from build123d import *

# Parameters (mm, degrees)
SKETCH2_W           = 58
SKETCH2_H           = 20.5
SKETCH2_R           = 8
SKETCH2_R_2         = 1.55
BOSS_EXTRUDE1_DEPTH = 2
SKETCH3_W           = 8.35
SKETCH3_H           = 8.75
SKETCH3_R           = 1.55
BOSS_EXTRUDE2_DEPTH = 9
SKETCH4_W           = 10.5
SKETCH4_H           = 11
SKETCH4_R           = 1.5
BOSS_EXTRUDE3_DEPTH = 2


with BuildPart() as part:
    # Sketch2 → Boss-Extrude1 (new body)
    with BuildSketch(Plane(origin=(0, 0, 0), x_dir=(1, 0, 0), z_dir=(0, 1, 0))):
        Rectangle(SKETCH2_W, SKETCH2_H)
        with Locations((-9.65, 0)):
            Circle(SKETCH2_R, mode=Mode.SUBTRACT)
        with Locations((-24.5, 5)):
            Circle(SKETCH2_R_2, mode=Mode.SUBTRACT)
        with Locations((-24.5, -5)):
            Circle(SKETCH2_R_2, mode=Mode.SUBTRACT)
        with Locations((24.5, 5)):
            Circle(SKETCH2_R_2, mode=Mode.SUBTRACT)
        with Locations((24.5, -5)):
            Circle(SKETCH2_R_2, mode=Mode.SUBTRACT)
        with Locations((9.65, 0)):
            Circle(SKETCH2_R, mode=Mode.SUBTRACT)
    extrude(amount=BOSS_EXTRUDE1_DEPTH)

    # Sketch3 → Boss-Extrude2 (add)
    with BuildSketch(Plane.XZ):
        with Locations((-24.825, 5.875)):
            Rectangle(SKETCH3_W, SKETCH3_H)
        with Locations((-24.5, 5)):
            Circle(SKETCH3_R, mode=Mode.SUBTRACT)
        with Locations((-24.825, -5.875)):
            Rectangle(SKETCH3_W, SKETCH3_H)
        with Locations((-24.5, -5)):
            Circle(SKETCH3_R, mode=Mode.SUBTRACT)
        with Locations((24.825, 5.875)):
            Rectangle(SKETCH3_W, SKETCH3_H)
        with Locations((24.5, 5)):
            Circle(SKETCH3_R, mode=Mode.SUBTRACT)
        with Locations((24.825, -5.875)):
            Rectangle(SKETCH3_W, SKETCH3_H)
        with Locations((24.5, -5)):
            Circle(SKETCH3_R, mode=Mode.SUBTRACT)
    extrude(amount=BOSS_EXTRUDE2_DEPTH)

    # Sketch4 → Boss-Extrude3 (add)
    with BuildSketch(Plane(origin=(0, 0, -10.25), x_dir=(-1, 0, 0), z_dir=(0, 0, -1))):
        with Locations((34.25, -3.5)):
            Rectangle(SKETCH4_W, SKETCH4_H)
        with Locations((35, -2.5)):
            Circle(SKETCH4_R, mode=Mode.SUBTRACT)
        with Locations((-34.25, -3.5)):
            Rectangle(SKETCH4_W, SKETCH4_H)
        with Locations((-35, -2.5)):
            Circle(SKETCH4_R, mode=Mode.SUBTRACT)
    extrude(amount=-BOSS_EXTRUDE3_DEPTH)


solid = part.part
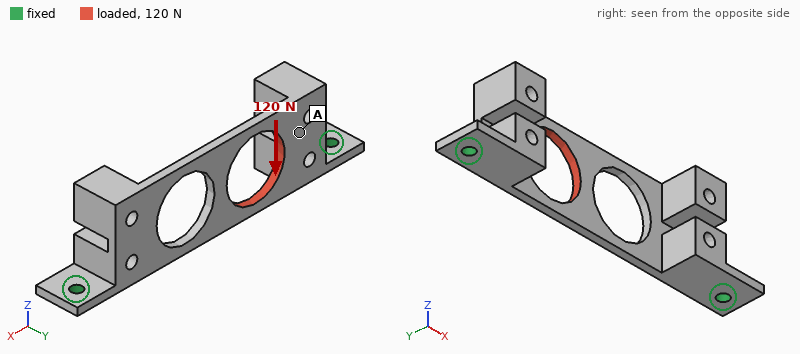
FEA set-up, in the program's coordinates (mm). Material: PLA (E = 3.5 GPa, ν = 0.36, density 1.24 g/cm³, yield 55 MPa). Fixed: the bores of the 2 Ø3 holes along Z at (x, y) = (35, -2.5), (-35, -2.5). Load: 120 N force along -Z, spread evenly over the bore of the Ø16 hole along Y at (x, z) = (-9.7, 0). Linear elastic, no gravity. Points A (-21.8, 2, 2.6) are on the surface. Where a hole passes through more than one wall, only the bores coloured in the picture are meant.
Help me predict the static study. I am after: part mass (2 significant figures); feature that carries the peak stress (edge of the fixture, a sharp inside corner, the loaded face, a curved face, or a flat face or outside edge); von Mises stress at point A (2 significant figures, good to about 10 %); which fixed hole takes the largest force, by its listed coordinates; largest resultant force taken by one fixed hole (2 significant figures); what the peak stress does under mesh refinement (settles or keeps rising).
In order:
5.3 g
edge of the fixture
6.7 MPa
(-35, -2.5)
90 N
keeps rising
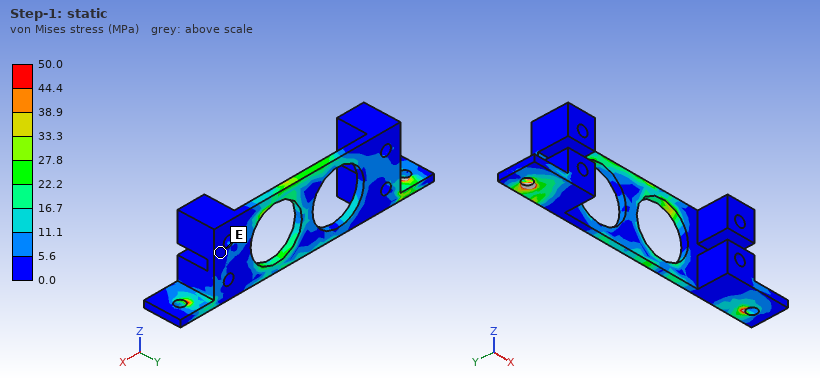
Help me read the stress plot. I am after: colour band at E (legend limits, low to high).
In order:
0.0 to 5.6 MPa
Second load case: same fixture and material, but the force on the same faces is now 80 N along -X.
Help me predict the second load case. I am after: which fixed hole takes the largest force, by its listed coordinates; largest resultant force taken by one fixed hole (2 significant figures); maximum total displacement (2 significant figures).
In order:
(-35, -2.5)
48 N
0.15 mm
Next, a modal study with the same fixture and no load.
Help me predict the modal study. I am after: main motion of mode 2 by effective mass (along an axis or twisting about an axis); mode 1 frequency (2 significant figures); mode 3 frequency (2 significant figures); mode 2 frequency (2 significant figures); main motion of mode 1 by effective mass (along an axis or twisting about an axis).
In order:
twisting about Z
670 Hz
1500 Hz
830 Hz
along Y
